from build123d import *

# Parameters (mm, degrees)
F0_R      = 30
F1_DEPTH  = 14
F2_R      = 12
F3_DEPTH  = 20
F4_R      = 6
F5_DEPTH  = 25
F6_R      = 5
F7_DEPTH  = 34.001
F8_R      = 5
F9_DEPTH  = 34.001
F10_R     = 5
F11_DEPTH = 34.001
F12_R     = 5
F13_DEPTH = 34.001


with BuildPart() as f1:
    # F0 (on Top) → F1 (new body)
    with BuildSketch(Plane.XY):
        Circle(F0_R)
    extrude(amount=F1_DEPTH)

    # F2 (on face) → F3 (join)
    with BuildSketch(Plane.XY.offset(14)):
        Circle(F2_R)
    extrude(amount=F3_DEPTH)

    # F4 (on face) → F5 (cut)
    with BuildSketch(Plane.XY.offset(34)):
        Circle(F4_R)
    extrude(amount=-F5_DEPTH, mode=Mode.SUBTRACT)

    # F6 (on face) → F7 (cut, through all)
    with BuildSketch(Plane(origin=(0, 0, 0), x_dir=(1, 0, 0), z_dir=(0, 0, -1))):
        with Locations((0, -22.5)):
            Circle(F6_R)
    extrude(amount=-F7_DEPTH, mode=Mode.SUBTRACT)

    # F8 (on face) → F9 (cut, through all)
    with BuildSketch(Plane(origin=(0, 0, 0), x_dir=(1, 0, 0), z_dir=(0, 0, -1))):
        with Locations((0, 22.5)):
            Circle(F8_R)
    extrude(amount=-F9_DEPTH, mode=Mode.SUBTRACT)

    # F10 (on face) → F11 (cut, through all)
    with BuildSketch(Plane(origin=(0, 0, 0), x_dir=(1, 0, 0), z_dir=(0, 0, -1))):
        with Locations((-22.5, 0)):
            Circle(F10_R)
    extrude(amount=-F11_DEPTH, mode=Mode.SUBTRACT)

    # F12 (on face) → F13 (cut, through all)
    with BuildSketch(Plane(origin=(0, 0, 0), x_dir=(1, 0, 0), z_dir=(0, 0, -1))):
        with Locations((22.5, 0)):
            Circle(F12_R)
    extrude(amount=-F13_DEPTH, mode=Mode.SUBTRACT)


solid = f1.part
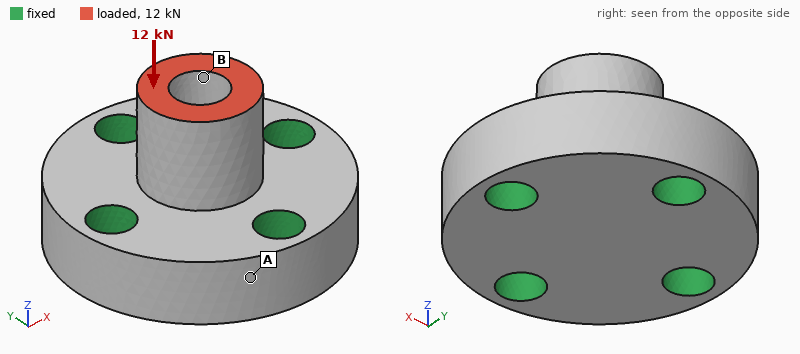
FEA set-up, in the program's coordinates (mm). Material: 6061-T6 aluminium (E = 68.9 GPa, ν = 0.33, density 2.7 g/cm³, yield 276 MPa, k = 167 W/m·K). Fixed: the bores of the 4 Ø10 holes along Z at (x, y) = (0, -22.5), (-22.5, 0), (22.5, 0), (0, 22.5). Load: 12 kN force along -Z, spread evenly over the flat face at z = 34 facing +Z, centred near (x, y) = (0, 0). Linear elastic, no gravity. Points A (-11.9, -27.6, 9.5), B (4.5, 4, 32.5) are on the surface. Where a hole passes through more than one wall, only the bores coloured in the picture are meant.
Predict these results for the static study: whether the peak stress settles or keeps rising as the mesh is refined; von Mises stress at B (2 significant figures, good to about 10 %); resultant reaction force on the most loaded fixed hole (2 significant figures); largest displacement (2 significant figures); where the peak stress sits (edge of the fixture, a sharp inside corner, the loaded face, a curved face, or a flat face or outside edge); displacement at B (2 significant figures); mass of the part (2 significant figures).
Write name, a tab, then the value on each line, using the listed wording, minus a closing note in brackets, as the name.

whether the peak stress settles or keeps rising as the mesh is refined	keeps rising
von Mises stress at B	36 MPa
resultant reaction force on the most loaded fixed hole	3.1 kN
largest displacement	17 µm
where the peak stress sits	edge of the fixture
displacement at B	16 µm
mass of the part	110 g
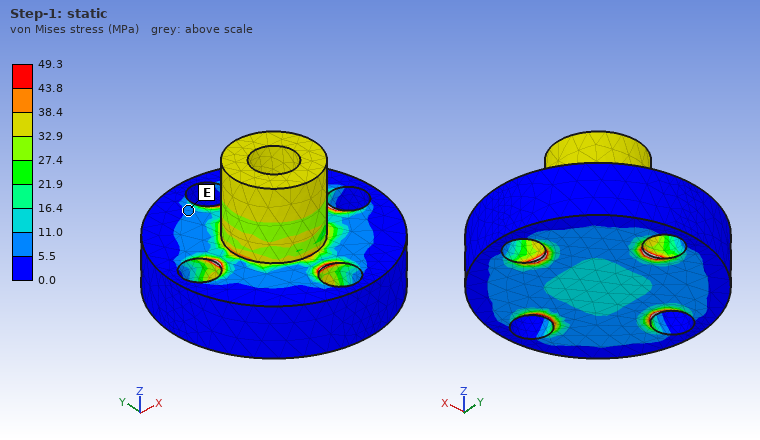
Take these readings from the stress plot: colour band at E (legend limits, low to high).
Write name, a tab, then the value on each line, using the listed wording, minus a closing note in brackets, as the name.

colour band at E	5.5 to 11.0 MPa
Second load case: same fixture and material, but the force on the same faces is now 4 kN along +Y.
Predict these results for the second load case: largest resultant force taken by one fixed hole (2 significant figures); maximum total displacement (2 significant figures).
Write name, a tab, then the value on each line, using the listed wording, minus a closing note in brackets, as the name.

largest resultant force taken by one fixed hole	3.0 kN
maximum total displacement	43 µm
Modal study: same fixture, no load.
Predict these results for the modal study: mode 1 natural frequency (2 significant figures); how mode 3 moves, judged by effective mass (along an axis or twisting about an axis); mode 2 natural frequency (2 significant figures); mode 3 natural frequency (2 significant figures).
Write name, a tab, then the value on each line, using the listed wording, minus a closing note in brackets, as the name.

mode 1 natural frequency	20 kHz
how mode 3 moves, judged by effective mass	along Z
mode 2 natural frequency	20 kHz
mode 3 natural frequency	32 kHz
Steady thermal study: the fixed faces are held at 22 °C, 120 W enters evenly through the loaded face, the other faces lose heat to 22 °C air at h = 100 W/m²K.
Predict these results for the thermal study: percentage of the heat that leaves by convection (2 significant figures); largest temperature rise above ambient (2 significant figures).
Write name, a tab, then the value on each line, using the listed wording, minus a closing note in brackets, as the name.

percentage of the heat that leaves by convection	6.9 %
largest temperature rise above ambient	52 K
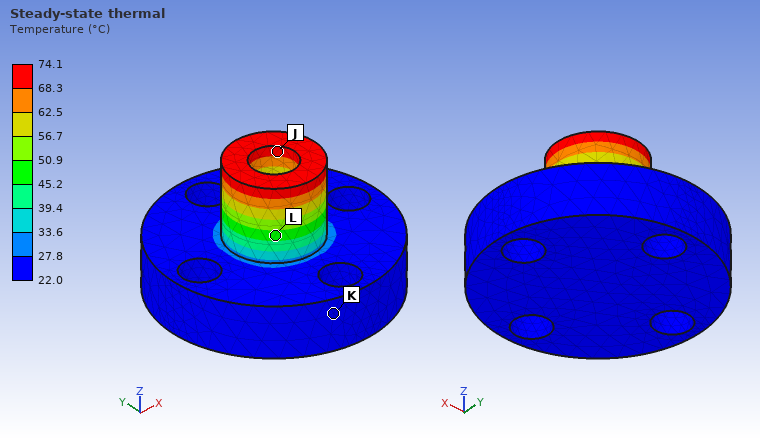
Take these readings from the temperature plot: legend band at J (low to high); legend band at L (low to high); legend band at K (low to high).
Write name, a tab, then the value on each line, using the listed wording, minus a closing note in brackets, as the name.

legend band at J	68.3 to 74.1 °C
legend band at L	45.2 to 50.9 °C
legend band at K	22.0 to 27.8 °C
